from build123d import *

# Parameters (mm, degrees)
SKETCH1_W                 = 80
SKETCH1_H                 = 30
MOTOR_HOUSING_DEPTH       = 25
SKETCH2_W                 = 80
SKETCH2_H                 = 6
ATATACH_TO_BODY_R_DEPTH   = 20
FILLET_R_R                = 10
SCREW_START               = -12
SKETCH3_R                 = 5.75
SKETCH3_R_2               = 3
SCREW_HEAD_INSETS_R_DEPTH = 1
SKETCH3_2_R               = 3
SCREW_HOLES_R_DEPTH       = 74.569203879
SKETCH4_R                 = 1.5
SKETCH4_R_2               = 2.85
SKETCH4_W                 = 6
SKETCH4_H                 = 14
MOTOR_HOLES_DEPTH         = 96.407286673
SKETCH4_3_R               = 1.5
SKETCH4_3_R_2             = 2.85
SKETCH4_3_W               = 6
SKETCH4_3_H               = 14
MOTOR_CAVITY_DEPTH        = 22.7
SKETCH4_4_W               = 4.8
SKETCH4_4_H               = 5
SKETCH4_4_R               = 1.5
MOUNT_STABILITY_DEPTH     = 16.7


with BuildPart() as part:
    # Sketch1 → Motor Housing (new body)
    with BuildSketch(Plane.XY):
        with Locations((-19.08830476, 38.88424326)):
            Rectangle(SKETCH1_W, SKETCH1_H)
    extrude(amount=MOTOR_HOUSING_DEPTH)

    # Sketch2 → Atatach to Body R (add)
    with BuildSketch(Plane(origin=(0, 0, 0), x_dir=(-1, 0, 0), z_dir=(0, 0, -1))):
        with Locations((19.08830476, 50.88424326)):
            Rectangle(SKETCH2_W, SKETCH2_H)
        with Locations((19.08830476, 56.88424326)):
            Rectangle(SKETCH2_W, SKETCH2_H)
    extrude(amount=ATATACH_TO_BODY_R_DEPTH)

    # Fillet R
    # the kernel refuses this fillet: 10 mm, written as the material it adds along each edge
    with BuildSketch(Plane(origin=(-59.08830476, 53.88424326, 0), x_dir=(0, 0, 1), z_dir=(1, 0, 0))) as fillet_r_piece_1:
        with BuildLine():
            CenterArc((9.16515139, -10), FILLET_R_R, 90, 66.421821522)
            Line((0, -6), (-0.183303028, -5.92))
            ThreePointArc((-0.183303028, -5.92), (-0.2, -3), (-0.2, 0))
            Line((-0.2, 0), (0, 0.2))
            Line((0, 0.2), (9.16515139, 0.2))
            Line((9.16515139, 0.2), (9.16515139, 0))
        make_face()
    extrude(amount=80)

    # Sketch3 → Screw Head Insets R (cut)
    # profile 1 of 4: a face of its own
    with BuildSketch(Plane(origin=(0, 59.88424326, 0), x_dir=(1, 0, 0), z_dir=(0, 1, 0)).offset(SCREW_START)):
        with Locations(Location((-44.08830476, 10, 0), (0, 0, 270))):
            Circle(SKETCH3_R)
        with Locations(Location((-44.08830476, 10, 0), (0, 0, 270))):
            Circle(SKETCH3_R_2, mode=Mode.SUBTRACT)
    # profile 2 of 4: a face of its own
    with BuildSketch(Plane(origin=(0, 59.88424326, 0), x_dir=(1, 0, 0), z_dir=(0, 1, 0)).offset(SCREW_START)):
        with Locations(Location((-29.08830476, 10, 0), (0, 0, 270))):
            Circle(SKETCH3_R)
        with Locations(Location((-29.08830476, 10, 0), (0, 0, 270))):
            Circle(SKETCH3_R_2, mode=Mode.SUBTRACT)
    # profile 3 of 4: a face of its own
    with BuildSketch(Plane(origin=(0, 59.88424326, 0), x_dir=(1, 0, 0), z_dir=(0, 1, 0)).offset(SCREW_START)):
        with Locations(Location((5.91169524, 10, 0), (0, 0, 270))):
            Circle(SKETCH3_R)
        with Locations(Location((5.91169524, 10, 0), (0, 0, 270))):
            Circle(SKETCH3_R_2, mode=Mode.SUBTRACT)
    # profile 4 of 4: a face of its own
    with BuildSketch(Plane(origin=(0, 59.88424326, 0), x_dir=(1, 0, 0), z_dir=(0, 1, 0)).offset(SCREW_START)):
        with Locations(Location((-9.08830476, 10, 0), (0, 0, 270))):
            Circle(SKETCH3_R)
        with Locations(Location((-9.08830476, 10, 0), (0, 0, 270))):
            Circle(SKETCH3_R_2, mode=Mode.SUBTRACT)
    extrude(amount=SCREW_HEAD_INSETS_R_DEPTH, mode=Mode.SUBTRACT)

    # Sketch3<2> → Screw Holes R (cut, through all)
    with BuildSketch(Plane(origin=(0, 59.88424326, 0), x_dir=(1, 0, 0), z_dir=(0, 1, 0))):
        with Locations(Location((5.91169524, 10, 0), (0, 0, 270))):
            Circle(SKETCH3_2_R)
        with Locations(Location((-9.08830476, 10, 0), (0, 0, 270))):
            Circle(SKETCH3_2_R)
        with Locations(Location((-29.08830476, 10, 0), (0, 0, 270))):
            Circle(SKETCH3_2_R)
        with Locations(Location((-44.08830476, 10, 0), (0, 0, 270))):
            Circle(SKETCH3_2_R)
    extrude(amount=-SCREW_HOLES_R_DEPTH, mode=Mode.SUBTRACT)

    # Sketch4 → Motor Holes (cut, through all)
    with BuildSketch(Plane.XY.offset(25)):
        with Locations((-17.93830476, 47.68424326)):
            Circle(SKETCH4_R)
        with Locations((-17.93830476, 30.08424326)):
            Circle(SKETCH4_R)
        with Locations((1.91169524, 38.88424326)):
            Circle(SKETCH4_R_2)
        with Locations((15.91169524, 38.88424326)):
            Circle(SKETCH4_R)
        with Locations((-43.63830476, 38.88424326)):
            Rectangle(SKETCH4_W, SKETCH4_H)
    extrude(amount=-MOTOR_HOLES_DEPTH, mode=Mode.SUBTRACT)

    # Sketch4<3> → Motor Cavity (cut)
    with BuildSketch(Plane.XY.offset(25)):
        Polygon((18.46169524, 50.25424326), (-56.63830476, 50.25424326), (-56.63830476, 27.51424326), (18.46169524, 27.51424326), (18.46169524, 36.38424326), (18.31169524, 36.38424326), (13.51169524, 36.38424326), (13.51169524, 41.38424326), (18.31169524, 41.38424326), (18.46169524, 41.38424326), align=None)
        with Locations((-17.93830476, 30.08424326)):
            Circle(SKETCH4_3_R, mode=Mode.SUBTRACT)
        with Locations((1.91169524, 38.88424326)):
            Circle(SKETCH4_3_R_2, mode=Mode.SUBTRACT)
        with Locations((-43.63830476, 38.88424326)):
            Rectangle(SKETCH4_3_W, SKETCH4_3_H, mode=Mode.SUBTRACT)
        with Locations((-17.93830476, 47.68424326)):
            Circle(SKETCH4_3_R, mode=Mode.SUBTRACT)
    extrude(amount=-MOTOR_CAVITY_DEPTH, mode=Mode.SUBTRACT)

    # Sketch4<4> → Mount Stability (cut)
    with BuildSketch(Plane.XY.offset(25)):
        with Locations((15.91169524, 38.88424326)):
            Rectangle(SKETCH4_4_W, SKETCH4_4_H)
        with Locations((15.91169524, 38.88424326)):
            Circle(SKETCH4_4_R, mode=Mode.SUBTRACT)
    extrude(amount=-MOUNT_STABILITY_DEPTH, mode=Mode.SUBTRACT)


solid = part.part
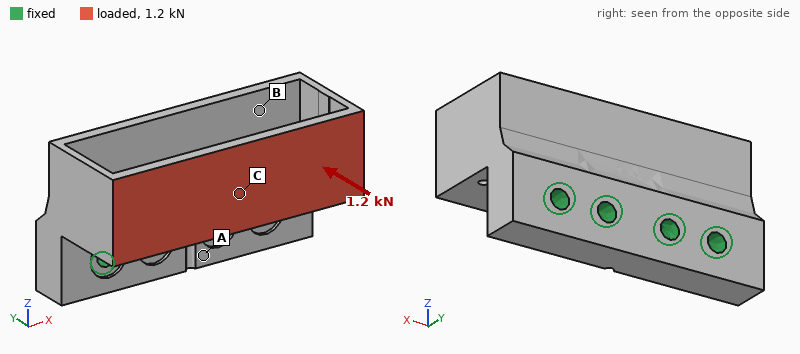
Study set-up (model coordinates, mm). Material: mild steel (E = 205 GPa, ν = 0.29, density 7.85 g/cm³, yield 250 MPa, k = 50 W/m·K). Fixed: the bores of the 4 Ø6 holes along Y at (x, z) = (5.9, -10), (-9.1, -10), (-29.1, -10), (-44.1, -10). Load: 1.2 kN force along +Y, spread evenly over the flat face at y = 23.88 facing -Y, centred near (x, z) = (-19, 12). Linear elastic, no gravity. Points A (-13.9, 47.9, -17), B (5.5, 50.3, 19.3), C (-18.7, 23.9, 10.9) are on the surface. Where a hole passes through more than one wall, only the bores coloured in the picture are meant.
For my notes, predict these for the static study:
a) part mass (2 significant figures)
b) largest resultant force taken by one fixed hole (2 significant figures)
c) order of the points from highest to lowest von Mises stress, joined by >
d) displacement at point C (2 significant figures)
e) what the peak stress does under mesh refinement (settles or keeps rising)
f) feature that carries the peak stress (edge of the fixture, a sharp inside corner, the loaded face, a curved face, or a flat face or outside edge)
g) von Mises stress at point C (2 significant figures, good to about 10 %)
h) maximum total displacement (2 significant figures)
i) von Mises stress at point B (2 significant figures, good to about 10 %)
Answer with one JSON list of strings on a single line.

["310 g", "330 N", "B > C > A", "42 µm", "keeps rising", "a sharp inside corner", "12 MPa", "79 µm", "17 MPa"]
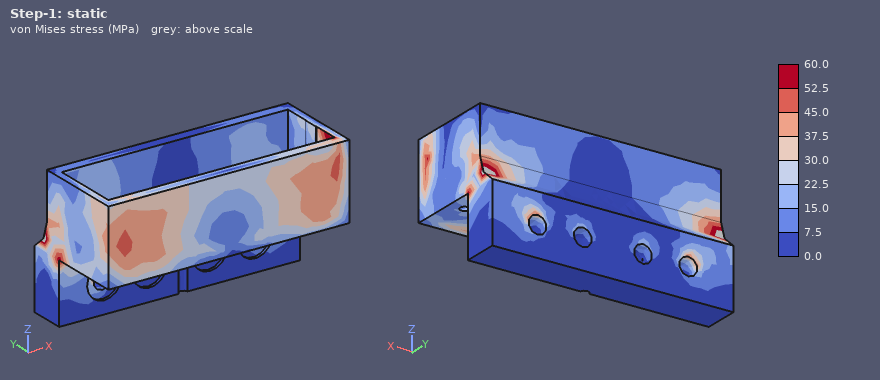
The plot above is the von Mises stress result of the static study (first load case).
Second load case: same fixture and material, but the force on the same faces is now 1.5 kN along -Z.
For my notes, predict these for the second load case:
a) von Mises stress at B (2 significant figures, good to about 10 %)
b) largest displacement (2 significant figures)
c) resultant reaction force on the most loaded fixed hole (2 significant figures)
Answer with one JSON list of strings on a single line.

["41 MPa", "0.11 mm", "760 N"]
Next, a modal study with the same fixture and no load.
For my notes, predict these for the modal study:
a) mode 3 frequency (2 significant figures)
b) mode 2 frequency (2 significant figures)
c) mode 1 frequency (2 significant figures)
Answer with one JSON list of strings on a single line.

["5100 Hz", "3700 Hz", "2500 Hz"]
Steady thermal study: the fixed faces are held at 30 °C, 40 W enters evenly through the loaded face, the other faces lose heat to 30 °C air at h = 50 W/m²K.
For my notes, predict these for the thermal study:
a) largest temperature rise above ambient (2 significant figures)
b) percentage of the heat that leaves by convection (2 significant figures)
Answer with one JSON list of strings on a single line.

["77 K", "46 %"]
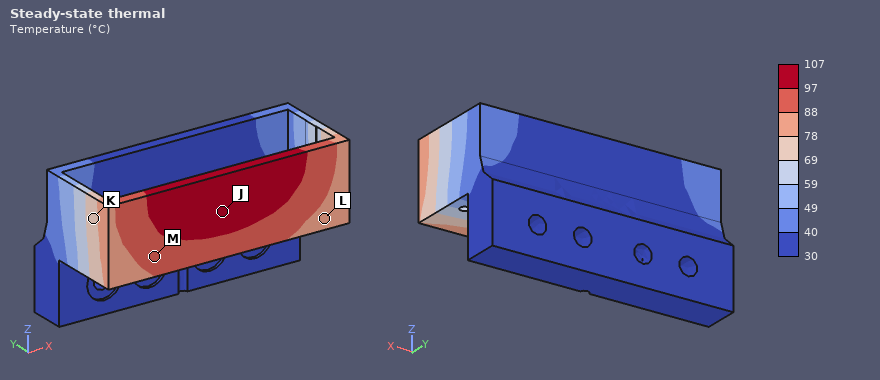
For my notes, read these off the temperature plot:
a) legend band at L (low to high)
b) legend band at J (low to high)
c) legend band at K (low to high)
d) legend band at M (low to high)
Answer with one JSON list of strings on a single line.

["78 to 88 °C", "97 to 107 °C", "69 to 78 °C", "88 to 97 °C"]
